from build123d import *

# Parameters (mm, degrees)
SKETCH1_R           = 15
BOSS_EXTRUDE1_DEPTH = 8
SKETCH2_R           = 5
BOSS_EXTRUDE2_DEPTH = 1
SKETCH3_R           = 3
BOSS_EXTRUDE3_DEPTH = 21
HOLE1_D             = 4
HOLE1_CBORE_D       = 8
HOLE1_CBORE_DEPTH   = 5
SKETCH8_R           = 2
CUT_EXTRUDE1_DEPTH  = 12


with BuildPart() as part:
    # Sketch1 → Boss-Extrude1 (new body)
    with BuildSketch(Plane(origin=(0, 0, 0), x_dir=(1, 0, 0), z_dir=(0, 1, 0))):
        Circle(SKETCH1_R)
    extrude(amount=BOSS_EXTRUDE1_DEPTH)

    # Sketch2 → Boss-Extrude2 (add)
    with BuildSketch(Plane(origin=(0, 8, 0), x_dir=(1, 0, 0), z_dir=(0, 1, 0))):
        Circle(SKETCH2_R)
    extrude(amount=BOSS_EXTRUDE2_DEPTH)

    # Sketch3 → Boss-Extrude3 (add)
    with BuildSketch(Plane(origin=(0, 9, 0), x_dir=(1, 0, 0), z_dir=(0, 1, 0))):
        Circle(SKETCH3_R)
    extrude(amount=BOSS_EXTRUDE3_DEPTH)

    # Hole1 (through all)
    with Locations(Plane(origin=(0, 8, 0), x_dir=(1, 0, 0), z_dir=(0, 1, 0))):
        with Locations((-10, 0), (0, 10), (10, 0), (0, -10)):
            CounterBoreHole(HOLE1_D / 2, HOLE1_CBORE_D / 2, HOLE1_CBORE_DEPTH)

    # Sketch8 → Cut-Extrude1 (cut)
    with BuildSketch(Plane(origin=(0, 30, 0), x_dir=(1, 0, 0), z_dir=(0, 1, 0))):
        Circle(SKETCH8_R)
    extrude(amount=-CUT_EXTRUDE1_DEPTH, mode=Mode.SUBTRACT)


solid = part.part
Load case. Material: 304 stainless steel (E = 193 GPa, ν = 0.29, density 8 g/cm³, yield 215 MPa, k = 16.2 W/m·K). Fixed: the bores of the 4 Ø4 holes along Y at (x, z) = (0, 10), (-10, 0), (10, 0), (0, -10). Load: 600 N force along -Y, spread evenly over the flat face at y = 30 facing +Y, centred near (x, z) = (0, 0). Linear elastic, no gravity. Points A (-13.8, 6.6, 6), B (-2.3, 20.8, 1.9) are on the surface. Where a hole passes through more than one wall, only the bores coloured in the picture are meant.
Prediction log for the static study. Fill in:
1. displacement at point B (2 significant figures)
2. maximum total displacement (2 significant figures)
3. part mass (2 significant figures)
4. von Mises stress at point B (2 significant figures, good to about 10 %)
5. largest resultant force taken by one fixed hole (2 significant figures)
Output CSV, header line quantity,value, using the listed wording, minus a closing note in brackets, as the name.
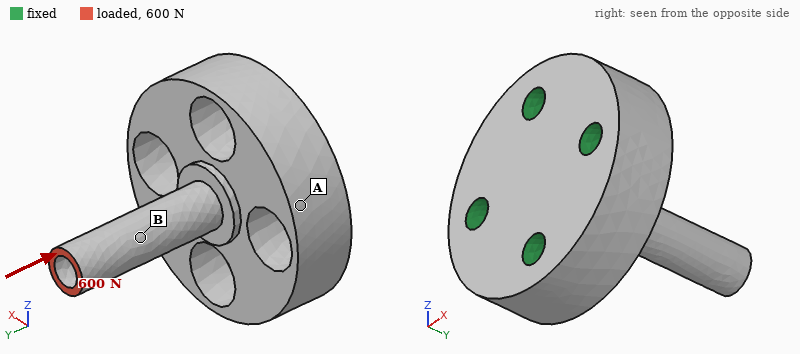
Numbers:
quantity,value
displacement at point B,2.3 µm
maximum total displacement,4.1 µm
part mass,40 g
von Mises stress at point B,39 MPa
largest resultant force taken by one fixed hole,160 N
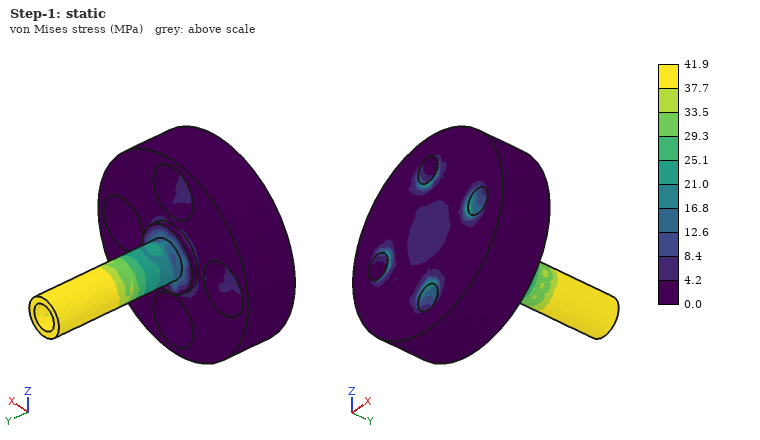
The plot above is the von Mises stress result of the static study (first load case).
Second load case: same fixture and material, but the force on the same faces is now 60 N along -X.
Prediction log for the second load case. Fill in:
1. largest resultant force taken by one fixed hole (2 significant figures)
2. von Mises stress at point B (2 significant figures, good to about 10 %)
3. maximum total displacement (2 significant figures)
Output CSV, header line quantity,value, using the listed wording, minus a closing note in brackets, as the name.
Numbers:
quantity,value
largest resultant force taken by one fixed hole,85 N
von Mises stress at point B,26 MPa
maximum total displacement,21 µm
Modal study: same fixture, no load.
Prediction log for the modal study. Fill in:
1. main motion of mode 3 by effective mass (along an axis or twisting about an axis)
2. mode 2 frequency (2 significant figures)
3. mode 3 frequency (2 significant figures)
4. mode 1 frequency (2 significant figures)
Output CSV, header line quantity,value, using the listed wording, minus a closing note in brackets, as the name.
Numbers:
quantity,value
main motion of mode 3 by effective mass,along X
mode 2 frequency,10 kHz
mode 3 frequency,37 kHz
mode 1 frequency,10 kHz
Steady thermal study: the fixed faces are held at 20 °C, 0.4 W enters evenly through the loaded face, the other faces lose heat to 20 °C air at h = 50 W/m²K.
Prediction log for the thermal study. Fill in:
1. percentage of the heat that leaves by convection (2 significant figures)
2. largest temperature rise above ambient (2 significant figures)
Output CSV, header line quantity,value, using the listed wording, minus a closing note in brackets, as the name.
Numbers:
quantity,value
percentage of the heat that leaves by convection,61 %
largest temperature rise above ambient,18 K
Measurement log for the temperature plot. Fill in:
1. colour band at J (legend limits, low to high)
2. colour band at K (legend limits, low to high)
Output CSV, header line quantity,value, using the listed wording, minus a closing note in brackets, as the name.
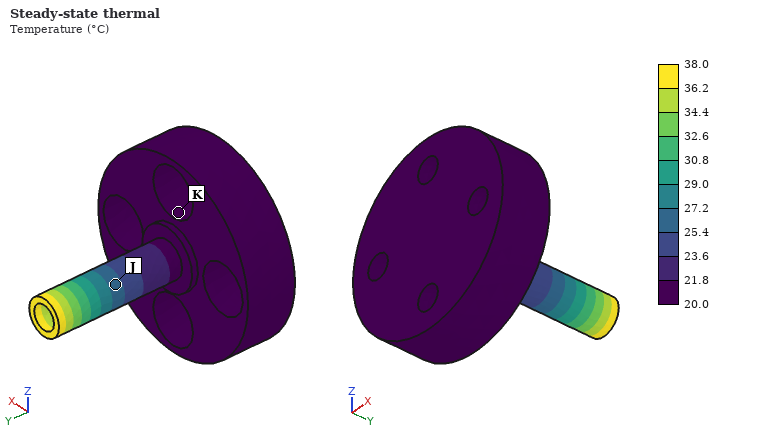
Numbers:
quantity,value
colour band at J,25.4 to 27.2 °C
colour band at K,20.0 to 21.8 °C
